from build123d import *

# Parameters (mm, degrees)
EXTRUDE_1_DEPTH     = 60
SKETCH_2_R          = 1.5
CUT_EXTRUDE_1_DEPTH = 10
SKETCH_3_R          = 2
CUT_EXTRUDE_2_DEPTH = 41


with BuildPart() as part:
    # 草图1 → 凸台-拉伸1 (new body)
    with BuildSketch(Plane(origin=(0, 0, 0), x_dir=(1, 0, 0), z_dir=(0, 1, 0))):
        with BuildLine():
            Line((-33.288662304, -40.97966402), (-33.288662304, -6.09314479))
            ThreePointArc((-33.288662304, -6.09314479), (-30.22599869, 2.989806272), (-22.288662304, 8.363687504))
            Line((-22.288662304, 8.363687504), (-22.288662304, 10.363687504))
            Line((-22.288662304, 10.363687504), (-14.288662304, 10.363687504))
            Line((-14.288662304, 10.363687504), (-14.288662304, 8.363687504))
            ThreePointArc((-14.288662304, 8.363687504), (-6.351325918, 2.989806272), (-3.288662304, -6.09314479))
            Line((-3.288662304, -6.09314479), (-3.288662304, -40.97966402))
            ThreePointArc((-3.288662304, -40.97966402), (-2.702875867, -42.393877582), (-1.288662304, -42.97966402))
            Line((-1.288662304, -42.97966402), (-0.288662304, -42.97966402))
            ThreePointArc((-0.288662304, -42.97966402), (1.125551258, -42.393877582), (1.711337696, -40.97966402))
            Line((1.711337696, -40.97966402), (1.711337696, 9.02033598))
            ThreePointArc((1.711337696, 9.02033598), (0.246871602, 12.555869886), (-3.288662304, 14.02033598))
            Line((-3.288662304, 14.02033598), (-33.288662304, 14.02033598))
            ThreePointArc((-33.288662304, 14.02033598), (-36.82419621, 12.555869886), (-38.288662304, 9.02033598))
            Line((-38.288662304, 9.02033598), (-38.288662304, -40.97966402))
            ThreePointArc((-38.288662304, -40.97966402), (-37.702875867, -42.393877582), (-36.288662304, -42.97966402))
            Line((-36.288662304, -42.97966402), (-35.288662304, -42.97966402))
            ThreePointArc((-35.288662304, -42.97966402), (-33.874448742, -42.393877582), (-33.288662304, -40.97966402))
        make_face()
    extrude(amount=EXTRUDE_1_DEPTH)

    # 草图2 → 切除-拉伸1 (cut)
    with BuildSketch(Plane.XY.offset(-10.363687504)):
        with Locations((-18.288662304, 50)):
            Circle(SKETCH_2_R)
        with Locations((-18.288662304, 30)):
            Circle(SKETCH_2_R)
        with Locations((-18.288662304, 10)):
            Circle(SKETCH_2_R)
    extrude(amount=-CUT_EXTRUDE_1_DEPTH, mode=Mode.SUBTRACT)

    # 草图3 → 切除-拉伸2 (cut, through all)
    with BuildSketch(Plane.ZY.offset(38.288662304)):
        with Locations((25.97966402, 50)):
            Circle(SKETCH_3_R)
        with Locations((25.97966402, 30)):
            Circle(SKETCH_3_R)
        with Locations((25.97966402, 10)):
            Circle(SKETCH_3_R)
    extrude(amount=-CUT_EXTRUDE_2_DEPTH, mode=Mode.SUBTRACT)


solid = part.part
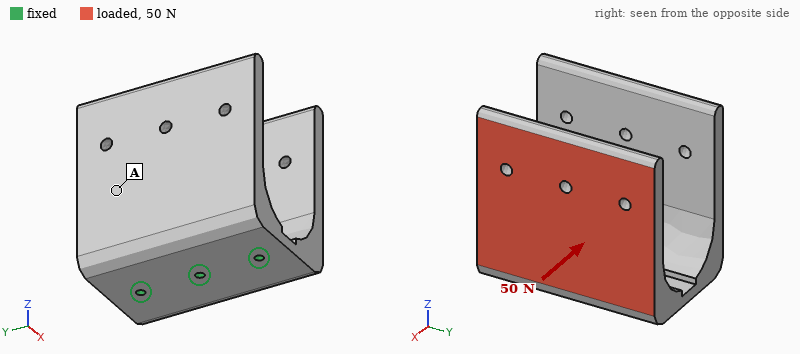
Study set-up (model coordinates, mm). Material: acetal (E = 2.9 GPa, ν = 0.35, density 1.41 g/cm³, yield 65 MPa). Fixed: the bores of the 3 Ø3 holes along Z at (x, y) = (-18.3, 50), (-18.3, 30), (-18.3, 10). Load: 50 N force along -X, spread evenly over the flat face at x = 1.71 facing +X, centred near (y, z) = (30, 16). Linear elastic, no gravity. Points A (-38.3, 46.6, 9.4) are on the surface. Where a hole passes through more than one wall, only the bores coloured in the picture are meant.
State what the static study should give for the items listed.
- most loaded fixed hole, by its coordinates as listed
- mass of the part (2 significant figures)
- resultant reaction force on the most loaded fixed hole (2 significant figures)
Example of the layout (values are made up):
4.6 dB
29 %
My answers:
(-18.3, 30)
66 g
21 N
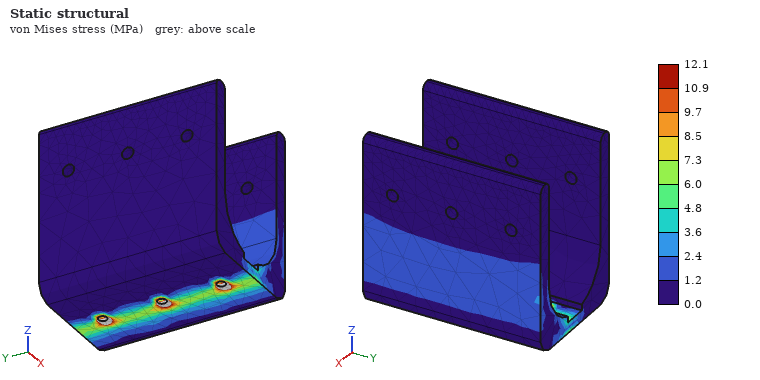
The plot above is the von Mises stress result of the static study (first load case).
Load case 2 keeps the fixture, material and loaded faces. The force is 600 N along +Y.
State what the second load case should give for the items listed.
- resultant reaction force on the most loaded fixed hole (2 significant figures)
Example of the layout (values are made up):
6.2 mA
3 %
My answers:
530 N
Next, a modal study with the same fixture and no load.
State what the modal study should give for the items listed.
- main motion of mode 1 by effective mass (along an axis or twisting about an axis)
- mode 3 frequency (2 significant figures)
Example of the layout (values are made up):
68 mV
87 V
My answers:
along X
760 Hz
